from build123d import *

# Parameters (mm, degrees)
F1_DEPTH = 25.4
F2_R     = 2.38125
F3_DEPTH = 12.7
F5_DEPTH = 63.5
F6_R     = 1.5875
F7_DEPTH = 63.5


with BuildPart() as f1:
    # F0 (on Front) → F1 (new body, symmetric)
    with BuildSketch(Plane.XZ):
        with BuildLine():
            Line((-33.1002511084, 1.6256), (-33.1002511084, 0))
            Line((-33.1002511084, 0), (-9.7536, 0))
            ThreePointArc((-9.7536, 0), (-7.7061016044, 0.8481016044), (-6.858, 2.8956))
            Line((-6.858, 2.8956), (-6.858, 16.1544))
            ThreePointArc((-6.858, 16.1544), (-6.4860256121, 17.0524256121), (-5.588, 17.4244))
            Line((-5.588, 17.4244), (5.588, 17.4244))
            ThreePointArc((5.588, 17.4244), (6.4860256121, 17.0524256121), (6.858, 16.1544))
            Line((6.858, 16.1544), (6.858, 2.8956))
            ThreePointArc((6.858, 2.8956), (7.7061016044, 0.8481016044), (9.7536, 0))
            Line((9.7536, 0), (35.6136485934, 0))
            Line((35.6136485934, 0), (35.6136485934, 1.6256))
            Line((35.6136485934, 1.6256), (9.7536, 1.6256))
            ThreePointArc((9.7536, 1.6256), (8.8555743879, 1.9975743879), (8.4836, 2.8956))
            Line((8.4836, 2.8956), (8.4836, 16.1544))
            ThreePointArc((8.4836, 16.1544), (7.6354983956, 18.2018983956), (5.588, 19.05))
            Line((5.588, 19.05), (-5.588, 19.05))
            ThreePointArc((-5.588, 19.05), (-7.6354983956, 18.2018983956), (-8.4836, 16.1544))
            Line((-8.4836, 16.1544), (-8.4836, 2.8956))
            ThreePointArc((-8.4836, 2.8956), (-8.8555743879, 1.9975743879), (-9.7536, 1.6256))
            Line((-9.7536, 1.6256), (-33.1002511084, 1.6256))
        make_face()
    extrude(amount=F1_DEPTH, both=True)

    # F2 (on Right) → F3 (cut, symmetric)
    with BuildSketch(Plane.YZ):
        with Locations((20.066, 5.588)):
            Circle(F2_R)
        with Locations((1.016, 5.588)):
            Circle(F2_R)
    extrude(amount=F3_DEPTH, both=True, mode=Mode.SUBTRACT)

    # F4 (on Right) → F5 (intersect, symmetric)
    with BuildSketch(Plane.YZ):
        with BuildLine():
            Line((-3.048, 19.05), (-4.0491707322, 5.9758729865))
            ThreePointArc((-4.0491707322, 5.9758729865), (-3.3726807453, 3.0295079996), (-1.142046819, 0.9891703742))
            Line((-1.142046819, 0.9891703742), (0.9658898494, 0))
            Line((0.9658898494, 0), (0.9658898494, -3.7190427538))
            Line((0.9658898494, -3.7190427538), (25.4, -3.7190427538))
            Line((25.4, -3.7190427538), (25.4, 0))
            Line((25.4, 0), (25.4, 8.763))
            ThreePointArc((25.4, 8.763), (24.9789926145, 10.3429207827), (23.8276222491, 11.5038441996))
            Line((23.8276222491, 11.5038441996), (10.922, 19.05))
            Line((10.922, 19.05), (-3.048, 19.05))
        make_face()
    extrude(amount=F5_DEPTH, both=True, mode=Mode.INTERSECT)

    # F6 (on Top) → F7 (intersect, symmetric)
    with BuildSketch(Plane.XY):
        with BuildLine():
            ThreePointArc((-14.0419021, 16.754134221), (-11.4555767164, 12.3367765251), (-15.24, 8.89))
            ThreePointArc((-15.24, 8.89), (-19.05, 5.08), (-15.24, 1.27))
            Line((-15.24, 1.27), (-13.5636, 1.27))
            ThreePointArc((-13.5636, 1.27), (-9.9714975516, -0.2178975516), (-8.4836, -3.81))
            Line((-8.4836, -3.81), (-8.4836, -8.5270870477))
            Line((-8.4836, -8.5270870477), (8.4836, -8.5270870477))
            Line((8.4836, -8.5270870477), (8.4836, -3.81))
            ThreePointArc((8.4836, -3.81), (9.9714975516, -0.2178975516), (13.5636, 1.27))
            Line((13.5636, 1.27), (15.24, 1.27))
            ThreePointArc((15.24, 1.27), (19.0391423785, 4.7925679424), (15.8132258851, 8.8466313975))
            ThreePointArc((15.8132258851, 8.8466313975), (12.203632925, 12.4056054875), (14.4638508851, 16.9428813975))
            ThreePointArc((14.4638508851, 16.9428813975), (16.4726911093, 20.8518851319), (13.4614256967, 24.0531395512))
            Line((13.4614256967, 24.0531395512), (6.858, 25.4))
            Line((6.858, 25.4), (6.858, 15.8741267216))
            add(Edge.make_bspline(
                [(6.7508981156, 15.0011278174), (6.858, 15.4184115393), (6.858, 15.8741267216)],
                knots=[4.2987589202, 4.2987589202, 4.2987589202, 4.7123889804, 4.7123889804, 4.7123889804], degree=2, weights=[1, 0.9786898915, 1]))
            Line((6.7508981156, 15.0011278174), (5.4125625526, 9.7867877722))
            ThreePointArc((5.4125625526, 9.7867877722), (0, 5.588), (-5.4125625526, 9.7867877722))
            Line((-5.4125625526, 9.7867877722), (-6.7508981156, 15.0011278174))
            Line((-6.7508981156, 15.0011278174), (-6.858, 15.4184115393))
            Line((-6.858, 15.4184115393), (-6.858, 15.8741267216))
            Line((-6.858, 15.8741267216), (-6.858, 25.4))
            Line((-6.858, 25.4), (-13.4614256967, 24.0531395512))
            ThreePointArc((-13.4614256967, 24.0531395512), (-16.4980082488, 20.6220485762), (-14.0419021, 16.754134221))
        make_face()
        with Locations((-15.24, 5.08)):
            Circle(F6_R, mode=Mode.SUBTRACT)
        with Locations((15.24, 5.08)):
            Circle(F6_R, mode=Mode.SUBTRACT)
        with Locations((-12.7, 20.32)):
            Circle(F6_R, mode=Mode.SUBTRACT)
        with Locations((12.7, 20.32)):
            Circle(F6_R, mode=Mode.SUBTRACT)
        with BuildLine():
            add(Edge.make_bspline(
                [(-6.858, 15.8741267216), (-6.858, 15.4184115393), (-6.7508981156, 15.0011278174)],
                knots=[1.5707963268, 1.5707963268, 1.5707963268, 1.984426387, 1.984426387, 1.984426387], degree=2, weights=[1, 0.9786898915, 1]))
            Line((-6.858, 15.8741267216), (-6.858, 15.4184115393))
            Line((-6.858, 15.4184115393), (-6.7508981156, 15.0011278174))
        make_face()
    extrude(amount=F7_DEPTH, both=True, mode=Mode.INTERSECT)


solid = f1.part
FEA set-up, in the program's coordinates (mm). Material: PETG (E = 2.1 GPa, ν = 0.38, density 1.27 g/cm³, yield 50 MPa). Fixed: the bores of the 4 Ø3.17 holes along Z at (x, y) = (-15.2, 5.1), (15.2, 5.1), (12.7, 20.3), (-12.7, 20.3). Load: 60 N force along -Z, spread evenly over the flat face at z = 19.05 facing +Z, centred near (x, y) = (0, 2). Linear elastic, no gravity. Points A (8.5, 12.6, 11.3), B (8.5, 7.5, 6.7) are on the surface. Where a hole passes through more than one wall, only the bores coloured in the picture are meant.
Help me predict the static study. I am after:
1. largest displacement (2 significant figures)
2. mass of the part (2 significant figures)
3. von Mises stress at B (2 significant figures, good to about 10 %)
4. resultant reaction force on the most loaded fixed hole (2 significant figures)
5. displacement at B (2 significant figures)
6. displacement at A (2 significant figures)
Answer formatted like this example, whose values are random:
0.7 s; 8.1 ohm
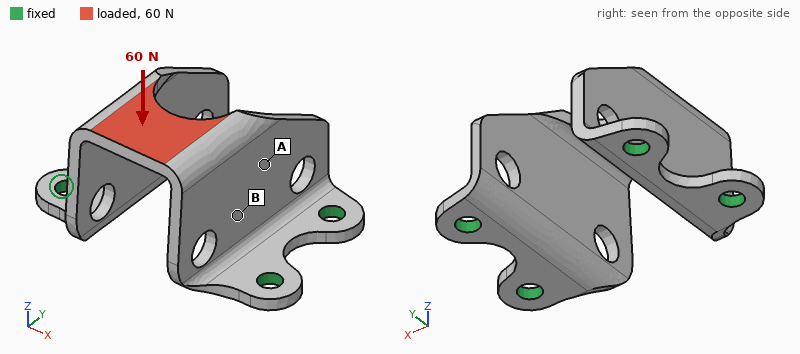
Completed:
0.55 mm; 2.6 g; 6.1 MPa; 34 N; 0.18 mm; 0.16 mm
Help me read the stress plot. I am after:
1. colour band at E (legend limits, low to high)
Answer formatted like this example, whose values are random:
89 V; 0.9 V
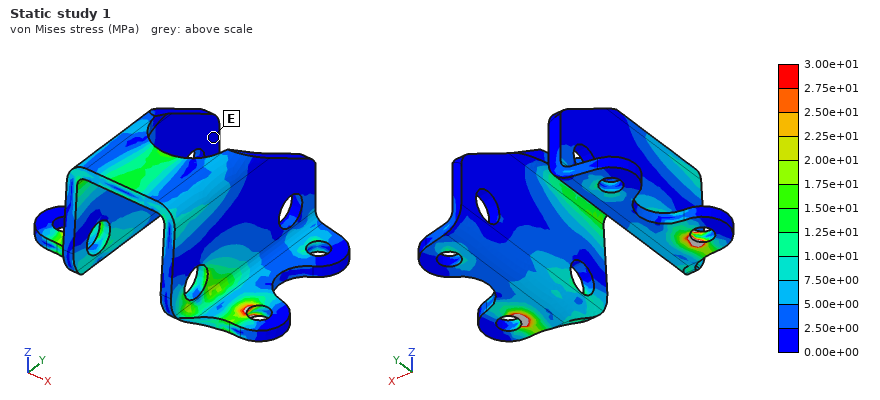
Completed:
0.00e+00 to 2.50e+00 MPa
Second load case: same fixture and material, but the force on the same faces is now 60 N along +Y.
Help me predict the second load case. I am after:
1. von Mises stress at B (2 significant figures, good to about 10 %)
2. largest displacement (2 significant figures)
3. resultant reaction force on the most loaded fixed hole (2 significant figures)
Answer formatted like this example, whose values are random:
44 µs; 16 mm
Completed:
5.5 MPa; 0.56 mm; 39 N
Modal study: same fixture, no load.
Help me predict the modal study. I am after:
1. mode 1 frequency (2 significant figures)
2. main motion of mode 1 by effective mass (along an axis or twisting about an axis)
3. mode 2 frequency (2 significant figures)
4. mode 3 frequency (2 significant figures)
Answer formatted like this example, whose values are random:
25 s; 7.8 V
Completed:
1000 Hz; along X; 1600 Hz; 1800 Hz
